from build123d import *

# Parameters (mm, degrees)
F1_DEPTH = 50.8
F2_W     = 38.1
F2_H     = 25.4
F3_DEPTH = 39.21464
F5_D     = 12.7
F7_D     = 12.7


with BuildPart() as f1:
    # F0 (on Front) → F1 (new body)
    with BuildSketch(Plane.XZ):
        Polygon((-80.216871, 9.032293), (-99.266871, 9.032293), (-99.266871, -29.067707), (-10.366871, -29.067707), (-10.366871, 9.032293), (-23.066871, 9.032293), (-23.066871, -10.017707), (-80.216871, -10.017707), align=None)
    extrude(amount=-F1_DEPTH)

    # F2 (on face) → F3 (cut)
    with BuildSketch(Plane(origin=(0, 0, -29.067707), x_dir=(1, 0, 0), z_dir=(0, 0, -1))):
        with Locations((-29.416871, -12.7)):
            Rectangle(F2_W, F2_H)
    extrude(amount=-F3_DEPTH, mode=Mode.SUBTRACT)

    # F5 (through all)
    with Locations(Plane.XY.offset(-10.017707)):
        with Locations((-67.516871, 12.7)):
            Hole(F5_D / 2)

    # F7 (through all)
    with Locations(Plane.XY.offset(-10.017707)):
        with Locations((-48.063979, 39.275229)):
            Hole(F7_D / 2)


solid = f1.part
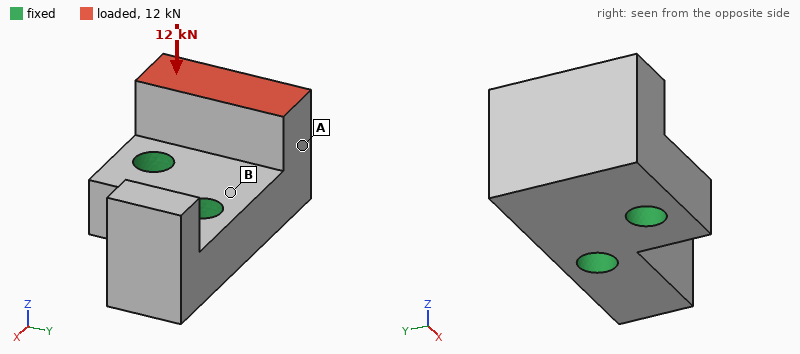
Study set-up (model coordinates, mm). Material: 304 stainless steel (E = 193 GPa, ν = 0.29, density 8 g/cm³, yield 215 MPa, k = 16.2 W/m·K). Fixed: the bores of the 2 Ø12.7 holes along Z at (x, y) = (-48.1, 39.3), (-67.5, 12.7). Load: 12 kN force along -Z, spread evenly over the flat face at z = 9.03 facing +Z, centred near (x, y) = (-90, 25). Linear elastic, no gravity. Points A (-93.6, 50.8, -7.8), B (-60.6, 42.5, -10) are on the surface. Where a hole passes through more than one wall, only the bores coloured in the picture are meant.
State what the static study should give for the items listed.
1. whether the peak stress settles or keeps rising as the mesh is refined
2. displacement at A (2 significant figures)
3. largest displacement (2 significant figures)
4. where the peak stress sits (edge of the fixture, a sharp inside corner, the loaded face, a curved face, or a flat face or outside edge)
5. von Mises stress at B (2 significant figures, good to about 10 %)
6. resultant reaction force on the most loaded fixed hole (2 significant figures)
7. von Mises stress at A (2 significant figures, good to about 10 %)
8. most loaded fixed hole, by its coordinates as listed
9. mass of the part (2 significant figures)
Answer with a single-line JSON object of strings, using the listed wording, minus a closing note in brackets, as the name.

{"whether the peak stress settles or keeps rising as the mesh is refined": "keeps rising", "displacement at A": "25 µm", "largest displacement": "35 µm", "where the peak stress sits": "edge of the fixture", "von Mises stress at B": "53 MPa", "resultant reaction force on the most loaded fixed hole": "10 kN", "von Mises stress at A": "11 MPa", "most loaded fixed hole, by its coordinates as listed": "(-67.5, 12.7)", "mass of the part": "700 g"}
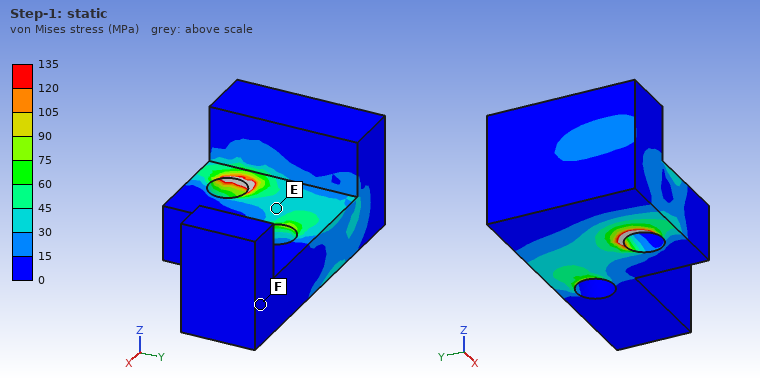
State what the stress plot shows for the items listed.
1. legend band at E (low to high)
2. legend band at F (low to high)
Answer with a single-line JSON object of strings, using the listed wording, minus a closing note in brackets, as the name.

{"legend band at E": "30 to 45 MPa", "legend band at F": "0 to 15 MPa"}
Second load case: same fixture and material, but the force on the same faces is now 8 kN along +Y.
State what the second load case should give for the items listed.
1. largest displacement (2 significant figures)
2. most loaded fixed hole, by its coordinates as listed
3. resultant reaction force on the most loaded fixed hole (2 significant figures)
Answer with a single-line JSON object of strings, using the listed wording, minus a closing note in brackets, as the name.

{"largest displacement": "29 µm", "most loaded fixed hole, by its coordinates as listed": "(-67.5, 12.7)", "resultant reaction force on the most loaded fixed hole": "9.5 kN"}
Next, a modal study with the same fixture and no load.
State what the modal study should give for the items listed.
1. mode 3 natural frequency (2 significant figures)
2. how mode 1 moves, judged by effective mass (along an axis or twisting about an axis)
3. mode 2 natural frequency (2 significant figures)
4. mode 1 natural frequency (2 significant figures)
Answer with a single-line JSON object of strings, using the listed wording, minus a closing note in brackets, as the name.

{"mode 3 natural frequency": "7100 Hz", "how mode 1 moves, judged by effective mass": "along Z", "mode 2 natural frequency": "6700 Hz", "mode 1 natural frequency": "6300 Hz"}
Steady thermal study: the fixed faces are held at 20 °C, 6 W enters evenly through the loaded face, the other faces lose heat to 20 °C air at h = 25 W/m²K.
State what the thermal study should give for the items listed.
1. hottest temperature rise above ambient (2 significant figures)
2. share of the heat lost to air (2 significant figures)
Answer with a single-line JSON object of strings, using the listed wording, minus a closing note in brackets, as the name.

{"hottest temperature rise above ambient": "15 K", "share of the heat lost to air": "21 %"}
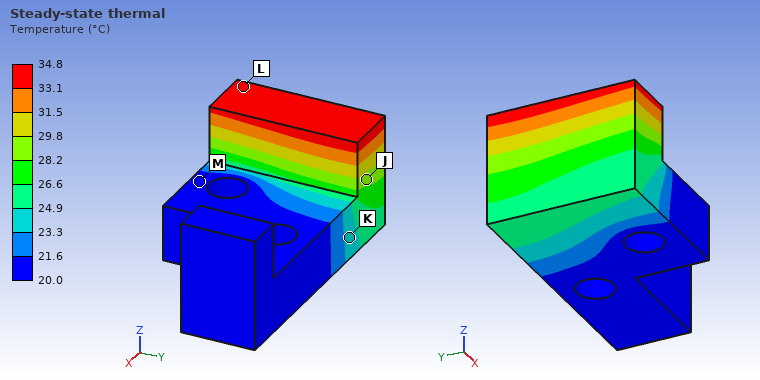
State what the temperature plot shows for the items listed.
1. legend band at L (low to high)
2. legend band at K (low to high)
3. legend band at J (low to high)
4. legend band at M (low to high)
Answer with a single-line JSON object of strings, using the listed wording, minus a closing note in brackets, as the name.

{"legend band at L": "33.1 to 34.8 °C", "legend band at K": "23.3 to 24.9 °C", "legend band at J": "28.2 to 29.8 °C", "legend band at M": "20.0 to 21.6 °C"}
